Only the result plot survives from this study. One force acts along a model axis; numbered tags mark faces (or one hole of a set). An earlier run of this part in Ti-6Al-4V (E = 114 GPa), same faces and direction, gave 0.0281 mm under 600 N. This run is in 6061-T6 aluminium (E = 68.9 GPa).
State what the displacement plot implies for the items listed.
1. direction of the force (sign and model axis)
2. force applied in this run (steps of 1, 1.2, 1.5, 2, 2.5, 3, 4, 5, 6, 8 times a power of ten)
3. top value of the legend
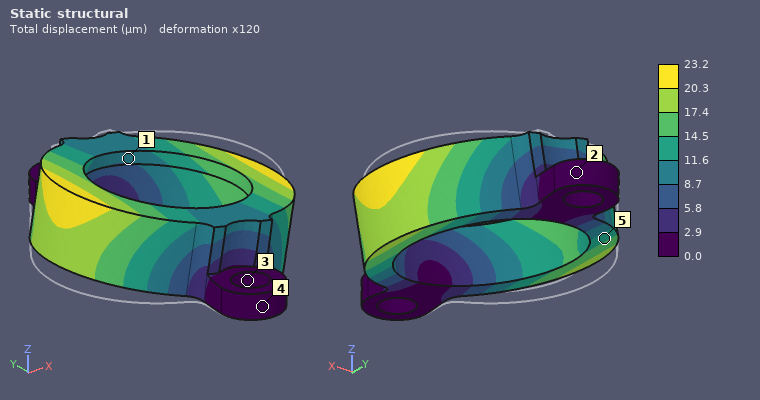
+X
300 N
23.2 µm
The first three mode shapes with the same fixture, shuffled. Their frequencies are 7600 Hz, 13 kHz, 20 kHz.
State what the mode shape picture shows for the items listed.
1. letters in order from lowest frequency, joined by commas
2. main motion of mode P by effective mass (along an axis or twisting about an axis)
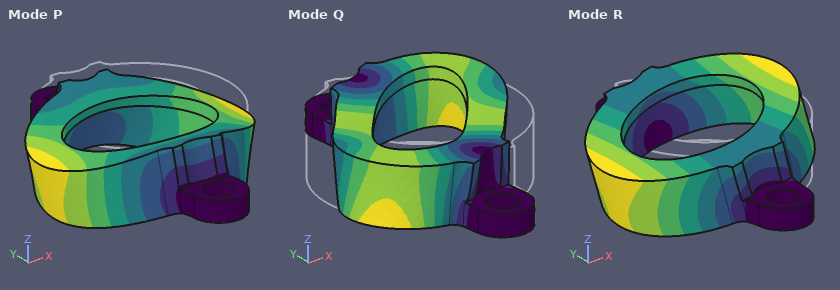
R, P, Q
along Z
